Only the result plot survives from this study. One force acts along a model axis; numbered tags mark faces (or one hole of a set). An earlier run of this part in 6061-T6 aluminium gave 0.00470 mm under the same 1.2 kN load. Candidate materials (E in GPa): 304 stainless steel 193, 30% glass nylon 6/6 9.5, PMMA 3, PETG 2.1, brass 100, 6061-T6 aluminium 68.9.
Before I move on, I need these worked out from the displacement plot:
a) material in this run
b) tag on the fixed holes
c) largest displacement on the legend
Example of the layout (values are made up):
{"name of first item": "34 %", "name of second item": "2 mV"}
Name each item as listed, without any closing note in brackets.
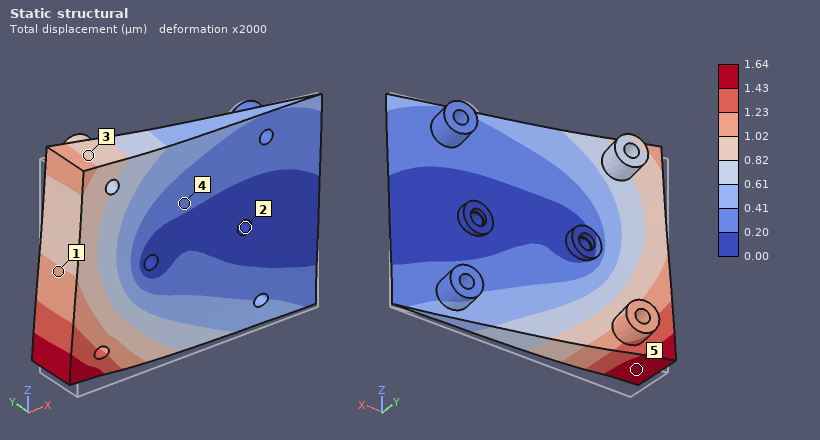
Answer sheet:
{"material in this run": "304 stainless steel", "tag on the fixed holes": "2", "largest displacement on the legend": "1.64 µm"}
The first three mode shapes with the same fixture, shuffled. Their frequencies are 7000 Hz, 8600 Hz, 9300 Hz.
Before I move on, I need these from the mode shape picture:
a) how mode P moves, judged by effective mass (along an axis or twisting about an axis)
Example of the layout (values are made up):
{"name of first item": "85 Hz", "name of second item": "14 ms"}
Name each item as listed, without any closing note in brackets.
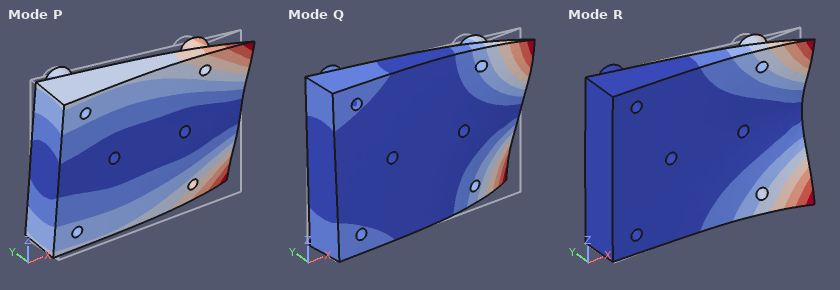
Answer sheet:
{"how mode P moves, judged by effective mass": "twisting about X"}
